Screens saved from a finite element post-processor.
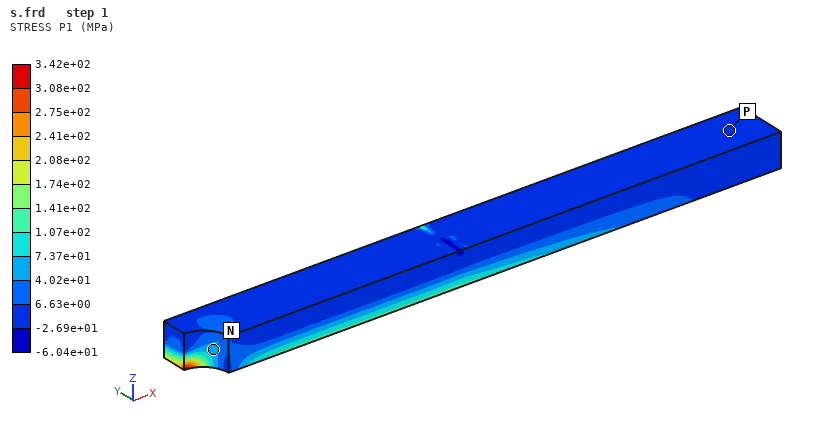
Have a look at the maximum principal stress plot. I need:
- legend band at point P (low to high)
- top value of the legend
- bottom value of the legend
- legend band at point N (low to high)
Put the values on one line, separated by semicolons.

-2.69e+01 to 6.63e+00 MPa; 3.42e+02 MPa; -6.04e+01 MPa; 4.02e+01 to 7.37e+01 MPa
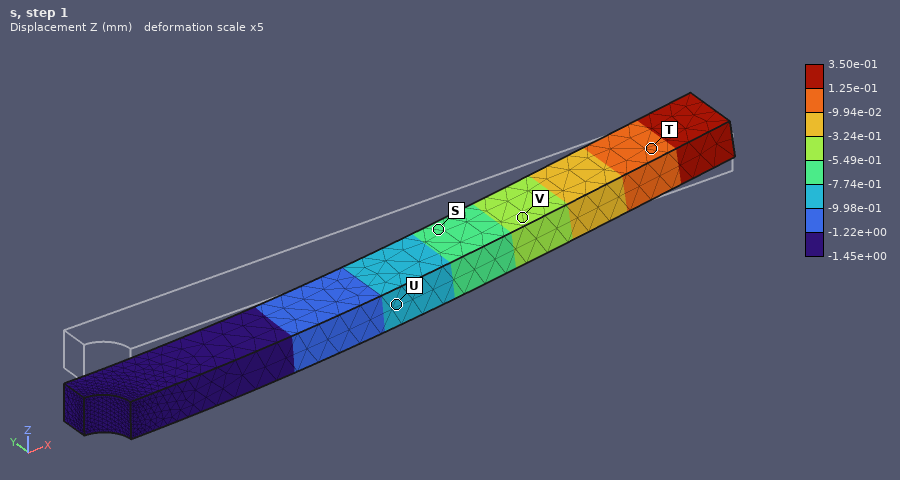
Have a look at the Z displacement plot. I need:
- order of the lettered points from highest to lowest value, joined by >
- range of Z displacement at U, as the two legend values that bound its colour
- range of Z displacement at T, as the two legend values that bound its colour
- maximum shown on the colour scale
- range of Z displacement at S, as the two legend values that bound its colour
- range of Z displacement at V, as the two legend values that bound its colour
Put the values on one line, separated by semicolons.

T > V > S > U; -9.98e-01 to -7.74e-01 mm; -9.94e-02 to 1.25e-01 mm; 3.50e-01 mm; -7.74e-01 to -5.49e-01 mm; -5.49e-01 to -3.24e-01 mm
